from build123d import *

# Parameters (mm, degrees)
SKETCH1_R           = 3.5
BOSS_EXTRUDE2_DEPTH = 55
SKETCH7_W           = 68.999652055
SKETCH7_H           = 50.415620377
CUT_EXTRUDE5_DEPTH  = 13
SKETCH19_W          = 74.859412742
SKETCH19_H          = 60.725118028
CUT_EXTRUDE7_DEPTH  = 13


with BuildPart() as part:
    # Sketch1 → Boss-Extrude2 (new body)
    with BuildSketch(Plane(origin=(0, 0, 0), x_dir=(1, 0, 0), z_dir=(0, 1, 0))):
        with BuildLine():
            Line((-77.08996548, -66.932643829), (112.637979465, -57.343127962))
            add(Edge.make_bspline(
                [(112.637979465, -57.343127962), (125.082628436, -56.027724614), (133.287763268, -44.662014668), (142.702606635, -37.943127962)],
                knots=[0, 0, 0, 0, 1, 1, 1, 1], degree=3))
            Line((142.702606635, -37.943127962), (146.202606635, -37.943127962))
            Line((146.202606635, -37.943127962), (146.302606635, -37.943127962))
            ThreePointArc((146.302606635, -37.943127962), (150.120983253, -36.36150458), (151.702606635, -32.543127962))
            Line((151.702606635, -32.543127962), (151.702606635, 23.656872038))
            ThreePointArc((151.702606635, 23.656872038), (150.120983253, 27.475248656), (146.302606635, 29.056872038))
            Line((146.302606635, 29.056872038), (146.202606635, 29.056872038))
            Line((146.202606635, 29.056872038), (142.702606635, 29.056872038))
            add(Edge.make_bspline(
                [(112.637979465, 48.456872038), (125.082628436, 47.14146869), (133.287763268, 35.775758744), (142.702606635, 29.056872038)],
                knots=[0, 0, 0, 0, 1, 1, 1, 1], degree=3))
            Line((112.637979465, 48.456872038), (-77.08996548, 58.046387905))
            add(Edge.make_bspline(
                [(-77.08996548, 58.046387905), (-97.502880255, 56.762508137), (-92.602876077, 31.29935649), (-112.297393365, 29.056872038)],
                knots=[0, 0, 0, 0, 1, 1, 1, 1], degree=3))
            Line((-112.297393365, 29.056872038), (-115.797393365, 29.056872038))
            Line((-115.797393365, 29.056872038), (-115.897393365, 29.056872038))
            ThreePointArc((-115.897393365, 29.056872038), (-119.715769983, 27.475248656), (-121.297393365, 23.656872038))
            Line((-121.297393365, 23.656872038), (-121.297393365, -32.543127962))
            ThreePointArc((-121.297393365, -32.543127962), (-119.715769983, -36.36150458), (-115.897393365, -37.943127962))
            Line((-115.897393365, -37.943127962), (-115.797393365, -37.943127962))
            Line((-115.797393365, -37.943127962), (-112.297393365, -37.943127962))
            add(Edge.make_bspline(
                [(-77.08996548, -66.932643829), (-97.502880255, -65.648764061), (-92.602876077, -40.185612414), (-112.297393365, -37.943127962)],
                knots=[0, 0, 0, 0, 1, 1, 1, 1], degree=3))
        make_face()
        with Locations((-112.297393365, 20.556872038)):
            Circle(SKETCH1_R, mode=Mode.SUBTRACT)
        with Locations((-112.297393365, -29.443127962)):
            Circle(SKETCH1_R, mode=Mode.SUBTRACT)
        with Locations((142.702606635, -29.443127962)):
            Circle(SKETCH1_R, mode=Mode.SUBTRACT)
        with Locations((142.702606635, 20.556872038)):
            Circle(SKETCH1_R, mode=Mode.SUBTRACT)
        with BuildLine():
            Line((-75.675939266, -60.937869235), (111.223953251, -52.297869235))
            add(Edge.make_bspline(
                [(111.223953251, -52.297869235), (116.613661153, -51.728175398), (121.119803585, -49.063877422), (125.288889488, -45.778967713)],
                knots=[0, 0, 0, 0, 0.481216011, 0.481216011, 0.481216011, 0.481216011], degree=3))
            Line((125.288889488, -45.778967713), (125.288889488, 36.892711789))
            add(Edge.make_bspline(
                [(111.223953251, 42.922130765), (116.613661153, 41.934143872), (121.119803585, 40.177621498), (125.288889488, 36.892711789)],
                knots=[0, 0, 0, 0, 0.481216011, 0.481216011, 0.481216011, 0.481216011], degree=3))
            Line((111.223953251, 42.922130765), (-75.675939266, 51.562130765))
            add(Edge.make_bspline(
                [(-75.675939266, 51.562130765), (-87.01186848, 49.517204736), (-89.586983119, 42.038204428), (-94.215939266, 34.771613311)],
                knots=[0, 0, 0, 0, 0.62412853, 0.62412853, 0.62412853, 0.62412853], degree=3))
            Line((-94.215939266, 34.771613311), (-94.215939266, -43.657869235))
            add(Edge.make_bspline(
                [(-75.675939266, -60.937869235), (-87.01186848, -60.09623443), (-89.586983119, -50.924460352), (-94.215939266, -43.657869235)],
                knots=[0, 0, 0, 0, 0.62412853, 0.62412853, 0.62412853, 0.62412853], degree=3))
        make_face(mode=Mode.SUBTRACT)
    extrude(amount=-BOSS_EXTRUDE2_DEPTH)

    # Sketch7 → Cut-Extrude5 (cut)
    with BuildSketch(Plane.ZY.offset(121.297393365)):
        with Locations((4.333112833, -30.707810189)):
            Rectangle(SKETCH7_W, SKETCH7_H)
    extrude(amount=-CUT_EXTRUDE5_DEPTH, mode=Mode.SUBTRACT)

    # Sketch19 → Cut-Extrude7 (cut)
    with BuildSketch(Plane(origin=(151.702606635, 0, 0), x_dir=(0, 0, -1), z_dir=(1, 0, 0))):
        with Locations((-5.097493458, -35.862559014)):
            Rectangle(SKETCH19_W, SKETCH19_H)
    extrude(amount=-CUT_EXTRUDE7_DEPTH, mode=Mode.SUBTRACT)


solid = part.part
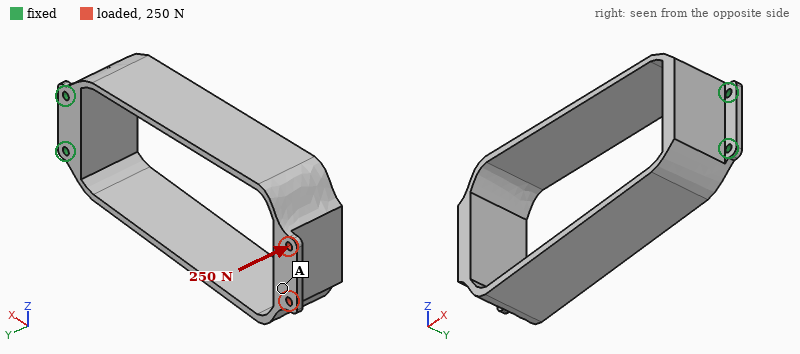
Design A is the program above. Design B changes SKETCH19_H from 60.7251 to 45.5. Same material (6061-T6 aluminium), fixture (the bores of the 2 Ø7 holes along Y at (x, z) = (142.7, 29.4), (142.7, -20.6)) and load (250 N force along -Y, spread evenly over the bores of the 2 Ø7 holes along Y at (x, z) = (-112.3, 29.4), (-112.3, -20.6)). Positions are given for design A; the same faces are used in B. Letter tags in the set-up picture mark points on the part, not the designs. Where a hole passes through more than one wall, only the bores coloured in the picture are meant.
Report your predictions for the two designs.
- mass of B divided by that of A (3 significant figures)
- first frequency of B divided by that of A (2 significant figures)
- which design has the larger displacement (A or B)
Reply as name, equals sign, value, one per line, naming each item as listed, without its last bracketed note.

mass of B divided by that of A = 1.02
first frequency of B divided by that of A = 1.0
which design has the larger displacement = A
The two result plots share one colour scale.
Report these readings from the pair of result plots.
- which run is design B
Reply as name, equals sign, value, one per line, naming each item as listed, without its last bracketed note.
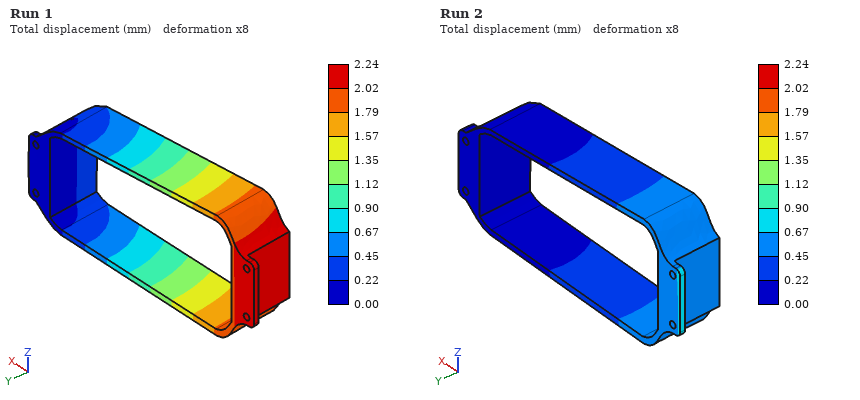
which run is design B = Run 2
